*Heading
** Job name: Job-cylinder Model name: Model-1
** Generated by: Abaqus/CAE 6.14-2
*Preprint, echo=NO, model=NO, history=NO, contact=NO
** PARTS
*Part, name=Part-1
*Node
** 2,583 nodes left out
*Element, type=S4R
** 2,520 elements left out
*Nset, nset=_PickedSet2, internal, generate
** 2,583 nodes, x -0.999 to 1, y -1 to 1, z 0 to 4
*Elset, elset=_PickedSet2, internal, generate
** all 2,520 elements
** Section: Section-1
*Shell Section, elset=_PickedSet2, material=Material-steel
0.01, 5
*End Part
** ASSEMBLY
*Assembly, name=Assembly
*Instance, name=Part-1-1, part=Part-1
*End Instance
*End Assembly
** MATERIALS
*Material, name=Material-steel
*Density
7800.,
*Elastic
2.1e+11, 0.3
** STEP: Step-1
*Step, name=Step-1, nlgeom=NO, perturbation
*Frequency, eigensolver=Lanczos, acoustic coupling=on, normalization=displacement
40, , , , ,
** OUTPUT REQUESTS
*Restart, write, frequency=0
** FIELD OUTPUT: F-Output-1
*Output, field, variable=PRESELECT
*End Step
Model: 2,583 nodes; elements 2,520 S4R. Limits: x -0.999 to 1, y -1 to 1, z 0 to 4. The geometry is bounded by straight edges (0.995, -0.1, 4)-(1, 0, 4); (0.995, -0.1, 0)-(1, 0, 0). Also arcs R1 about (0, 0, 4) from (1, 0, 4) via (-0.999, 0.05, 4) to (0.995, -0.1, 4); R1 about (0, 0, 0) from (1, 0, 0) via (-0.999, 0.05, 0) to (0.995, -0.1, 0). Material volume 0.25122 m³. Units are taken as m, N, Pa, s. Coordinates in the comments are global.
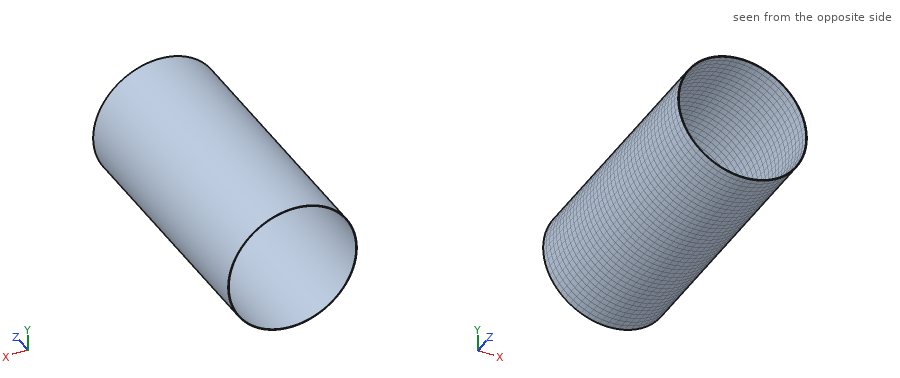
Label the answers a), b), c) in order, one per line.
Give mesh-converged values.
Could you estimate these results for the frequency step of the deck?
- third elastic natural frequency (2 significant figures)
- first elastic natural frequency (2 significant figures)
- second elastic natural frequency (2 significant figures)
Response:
a) 7.4 Hz
b) 6.7 Hz
c) 6.7 Hz
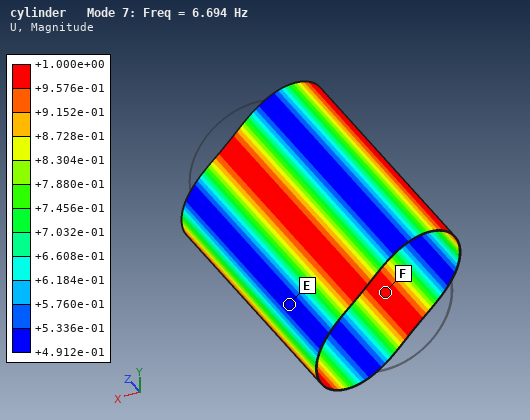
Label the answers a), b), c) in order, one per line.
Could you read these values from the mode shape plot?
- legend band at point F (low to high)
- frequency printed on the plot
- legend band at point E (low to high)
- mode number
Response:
a) +9.576e-01 to +1.000e+00
b) 6.694 Hz
c) +4.912e-01 to +5.336e-01
d) 7
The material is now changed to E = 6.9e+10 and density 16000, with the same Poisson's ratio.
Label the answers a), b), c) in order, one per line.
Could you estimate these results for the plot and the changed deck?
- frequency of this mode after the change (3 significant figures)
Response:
a) 2.68 Hz
